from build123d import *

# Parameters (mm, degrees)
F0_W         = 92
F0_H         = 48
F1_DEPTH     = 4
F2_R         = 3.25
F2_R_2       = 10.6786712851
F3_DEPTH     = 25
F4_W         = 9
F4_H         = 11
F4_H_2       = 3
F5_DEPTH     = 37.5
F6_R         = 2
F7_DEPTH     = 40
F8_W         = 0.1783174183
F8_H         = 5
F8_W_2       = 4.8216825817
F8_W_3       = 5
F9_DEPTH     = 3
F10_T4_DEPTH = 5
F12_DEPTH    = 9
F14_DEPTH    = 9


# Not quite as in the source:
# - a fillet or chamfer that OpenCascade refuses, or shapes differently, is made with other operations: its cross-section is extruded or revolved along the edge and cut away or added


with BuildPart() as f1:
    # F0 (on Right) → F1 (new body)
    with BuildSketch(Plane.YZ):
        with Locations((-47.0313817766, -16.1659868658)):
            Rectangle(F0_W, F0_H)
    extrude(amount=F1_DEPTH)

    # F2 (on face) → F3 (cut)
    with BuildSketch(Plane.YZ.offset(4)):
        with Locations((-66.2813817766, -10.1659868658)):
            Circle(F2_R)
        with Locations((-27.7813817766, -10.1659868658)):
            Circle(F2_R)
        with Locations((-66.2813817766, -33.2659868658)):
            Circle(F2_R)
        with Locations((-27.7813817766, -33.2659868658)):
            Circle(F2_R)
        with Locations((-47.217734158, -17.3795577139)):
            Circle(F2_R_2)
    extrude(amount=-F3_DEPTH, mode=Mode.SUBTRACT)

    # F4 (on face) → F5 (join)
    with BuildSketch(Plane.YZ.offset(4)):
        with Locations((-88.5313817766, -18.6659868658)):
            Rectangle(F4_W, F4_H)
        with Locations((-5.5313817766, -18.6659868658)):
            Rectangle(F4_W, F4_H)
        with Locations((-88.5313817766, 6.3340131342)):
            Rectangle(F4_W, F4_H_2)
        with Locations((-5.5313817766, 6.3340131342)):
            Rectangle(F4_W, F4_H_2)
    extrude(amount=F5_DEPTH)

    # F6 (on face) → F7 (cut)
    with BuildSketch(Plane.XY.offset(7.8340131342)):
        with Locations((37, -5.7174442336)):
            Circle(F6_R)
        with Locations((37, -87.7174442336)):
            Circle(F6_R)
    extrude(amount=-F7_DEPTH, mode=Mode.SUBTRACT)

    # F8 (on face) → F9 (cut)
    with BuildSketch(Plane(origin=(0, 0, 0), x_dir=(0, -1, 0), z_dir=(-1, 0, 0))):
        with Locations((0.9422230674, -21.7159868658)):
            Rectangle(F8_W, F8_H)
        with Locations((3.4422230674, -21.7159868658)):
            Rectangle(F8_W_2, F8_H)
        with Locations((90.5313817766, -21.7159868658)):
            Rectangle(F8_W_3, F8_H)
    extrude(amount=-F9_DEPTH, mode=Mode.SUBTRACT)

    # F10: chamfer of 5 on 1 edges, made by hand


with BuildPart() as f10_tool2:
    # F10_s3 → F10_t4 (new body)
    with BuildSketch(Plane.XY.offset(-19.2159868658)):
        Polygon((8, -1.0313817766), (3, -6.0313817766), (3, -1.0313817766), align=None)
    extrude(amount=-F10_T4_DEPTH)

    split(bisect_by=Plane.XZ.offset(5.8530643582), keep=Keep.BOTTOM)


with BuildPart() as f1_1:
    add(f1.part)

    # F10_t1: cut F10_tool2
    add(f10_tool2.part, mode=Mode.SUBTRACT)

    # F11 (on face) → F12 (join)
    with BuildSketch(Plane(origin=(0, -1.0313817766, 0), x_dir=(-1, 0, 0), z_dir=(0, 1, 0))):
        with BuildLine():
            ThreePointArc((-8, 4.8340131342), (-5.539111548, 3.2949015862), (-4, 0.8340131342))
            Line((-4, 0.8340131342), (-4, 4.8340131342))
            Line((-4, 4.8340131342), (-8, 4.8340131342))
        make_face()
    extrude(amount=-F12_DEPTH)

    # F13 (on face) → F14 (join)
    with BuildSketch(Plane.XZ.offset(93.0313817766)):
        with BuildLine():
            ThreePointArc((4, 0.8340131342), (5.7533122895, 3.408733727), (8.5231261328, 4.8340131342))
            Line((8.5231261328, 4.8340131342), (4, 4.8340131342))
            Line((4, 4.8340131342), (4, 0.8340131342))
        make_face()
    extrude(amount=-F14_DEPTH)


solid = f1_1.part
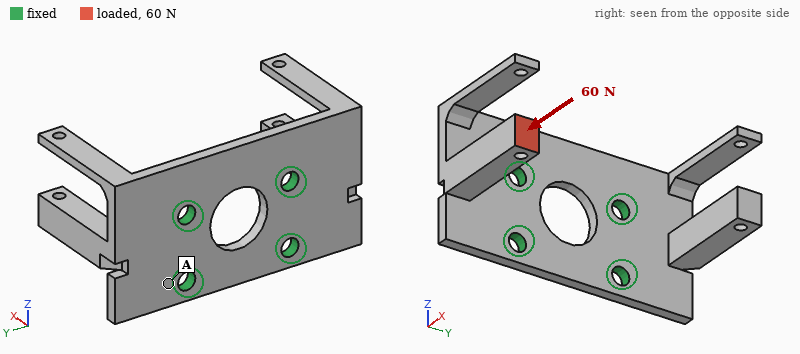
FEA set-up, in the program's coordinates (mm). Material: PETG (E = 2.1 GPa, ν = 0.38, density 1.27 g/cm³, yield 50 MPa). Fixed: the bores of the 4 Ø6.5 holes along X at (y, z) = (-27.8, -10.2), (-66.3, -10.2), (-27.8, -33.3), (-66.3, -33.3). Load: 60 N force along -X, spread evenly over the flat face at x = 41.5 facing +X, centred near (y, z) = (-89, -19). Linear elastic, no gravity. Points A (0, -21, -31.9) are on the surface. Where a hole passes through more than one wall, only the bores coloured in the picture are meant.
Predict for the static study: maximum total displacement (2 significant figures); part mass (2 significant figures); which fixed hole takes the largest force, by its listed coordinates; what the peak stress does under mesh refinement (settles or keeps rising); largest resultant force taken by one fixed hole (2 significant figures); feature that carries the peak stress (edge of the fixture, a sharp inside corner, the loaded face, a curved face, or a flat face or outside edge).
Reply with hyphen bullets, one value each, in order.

- 1.1 mm
- 31 g
- (-66.3, -10.2)
- keeps rising
- 39 N
- edge of the fixture
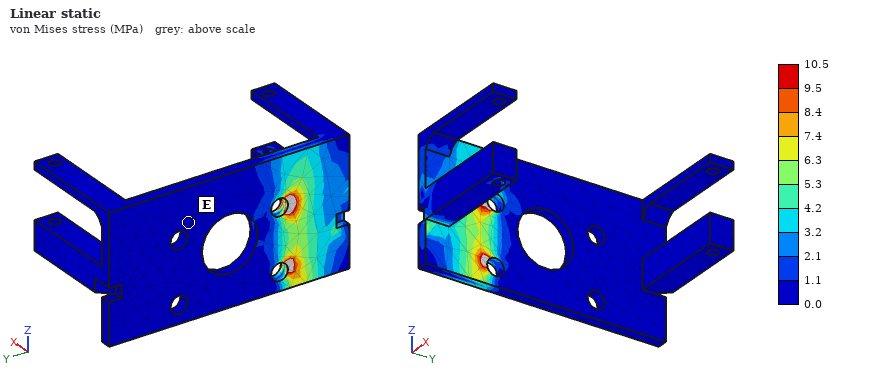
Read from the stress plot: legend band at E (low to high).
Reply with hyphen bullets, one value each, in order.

- 0.0 to 1.1 MPa
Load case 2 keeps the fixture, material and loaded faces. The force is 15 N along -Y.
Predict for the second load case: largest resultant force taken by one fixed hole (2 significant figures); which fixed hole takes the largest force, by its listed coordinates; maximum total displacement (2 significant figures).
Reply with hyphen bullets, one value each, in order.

- 13 N
- (-66.3, -10.2)
- 1.2 mm
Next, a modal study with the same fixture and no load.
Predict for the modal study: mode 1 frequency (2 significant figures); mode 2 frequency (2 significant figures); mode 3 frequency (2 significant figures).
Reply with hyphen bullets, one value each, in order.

- 380 Hz
- 390 Hz
- 420 Hz
